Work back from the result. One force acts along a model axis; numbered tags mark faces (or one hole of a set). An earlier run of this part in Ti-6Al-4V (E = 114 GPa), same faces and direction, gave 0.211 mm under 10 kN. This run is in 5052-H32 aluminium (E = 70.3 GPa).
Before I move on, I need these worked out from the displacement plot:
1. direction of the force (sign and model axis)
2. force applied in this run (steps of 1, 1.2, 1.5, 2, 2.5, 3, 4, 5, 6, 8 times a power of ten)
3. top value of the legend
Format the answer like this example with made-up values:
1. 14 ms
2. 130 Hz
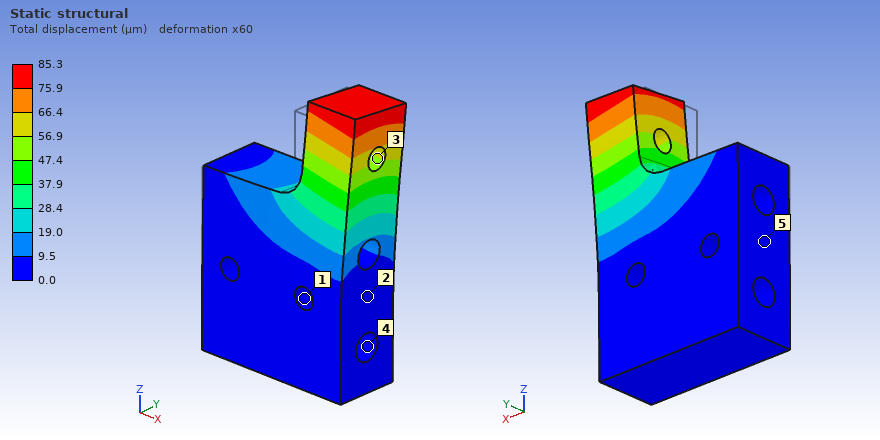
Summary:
1. +Y
2. 2.5 kN
3. 85.3 µm
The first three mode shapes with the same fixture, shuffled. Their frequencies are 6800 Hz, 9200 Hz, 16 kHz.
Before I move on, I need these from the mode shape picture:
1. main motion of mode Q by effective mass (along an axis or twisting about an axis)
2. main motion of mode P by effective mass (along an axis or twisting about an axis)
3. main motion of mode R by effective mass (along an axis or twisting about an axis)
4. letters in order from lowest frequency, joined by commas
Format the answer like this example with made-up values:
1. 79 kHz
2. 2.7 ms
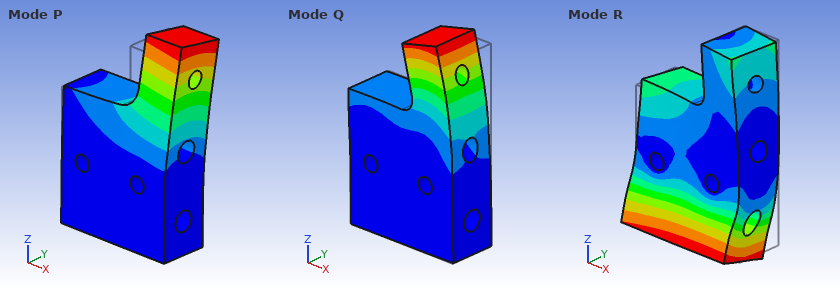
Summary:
1. along X
2. along Y
3. along Y
4. P, Q, R
